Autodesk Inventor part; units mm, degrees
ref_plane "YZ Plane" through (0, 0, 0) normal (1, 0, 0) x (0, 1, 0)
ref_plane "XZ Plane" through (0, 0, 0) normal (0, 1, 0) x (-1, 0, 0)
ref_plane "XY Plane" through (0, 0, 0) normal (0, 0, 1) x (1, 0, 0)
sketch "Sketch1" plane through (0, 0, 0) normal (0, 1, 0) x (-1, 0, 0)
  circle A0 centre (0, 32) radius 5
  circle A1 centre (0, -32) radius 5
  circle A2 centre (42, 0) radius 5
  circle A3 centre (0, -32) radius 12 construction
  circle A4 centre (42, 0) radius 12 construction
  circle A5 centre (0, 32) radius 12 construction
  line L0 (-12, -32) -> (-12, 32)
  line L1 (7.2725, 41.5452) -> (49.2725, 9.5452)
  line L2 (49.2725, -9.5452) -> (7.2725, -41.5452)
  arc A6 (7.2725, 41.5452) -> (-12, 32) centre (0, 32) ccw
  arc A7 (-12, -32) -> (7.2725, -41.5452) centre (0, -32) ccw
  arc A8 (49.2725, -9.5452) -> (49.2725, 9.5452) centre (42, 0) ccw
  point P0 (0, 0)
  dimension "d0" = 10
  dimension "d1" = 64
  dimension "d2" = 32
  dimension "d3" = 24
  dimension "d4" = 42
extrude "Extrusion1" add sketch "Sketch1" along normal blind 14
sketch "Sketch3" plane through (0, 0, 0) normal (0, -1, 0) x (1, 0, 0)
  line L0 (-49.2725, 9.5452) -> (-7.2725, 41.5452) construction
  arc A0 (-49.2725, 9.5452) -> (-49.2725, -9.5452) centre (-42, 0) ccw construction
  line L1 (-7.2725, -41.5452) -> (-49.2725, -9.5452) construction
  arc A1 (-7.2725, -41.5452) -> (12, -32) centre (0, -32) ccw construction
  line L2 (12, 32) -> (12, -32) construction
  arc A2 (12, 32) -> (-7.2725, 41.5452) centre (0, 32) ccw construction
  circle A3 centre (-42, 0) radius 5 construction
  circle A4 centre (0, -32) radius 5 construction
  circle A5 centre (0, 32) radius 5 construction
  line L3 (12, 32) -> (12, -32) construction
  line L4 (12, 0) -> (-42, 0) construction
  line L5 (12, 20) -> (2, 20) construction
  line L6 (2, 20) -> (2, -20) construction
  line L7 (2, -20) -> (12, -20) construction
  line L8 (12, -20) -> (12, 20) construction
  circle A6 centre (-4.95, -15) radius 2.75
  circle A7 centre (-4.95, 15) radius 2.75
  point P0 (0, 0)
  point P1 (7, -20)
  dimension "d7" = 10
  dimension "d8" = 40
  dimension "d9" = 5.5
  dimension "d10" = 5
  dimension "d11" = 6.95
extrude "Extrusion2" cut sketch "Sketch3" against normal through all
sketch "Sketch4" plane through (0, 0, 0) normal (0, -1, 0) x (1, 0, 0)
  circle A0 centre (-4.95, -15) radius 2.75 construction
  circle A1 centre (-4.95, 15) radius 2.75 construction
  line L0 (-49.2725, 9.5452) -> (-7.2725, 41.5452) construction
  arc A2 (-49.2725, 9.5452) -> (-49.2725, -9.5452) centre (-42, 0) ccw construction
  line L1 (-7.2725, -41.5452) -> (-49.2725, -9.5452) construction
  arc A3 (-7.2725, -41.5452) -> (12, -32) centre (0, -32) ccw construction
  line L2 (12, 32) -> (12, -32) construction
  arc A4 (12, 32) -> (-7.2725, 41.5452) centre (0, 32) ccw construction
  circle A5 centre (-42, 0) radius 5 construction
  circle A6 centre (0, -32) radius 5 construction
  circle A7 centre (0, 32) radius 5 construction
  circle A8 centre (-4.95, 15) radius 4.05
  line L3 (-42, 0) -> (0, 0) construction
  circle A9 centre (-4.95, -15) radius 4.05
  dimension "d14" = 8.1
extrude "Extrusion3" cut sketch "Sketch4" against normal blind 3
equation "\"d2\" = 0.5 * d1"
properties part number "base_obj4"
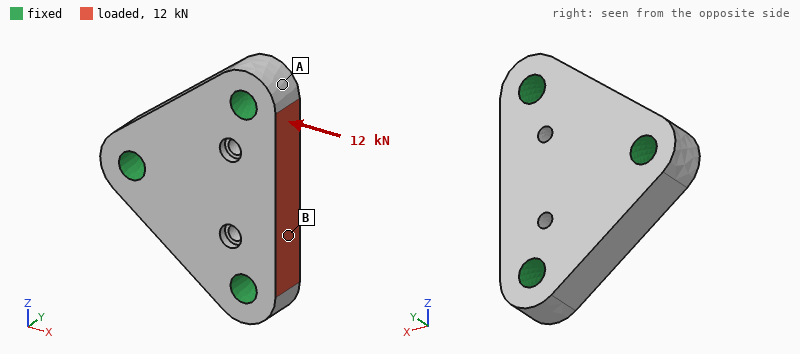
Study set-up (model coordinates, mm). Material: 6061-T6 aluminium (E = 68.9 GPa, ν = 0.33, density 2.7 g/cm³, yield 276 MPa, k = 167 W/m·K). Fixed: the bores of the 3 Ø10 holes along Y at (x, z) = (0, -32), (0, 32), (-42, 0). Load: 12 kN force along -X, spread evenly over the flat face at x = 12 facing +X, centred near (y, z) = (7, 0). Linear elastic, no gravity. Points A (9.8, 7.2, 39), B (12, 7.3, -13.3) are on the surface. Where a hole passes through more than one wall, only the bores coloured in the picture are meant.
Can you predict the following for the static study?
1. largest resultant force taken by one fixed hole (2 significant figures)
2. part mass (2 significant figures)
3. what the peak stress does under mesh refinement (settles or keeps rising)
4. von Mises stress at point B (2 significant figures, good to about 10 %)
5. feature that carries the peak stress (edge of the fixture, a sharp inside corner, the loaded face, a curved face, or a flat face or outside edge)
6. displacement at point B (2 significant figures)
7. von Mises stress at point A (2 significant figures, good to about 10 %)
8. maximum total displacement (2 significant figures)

4.3 kN
130 g
keeps rising
14 MPa
edge of the fixture
7.8 µm
4.5 MPa
9.1 µm
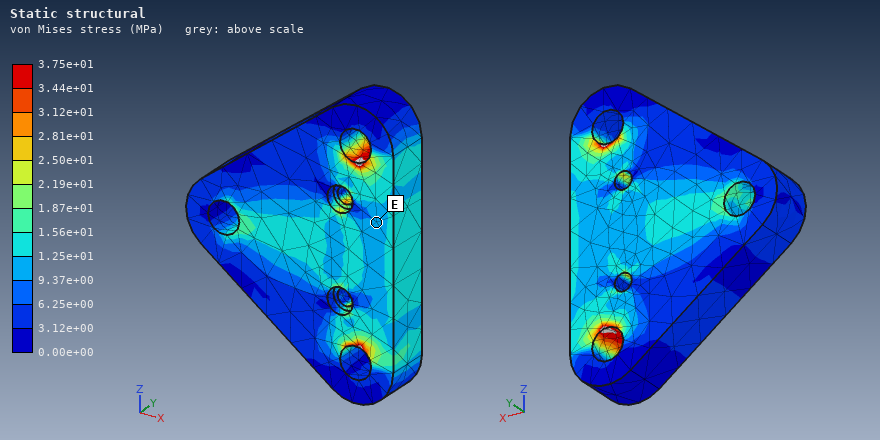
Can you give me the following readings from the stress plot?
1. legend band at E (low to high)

9.37e+00 to 1.25e+01 MPa
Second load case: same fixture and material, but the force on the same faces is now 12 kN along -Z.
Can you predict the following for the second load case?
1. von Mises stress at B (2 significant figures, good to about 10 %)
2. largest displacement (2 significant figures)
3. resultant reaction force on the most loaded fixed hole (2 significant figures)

25 MPa
8.3 µm
6.2 kN
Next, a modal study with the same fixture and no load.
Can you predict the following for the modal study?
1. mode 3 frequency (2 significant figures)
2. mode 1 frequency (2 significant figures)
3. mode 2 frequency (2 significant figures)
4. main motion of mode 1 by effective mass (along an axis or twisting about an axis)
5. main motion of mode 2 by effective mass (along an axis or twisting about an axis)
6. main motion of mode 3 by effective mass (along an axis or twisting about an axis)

23 kHz
16 kHz
22 kHz
along Y
along Y
twisting about X
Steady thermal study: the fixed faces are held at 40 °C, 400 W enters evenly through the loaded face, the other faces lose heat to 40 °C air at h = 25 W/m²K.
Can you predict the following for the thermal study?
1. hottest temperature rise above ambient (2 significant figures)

63 K
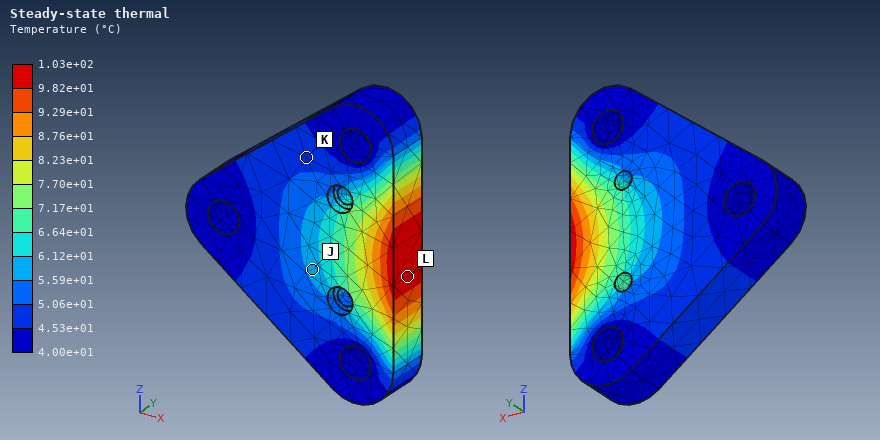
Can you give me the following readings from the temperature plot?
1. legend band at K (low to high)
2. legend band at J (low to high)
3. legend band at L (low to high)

4.53e+01 to 5.06e+01 °C
5.59e+01 to 6.12e+01 °C
9.82e+01 to 1.03e+02 °C
